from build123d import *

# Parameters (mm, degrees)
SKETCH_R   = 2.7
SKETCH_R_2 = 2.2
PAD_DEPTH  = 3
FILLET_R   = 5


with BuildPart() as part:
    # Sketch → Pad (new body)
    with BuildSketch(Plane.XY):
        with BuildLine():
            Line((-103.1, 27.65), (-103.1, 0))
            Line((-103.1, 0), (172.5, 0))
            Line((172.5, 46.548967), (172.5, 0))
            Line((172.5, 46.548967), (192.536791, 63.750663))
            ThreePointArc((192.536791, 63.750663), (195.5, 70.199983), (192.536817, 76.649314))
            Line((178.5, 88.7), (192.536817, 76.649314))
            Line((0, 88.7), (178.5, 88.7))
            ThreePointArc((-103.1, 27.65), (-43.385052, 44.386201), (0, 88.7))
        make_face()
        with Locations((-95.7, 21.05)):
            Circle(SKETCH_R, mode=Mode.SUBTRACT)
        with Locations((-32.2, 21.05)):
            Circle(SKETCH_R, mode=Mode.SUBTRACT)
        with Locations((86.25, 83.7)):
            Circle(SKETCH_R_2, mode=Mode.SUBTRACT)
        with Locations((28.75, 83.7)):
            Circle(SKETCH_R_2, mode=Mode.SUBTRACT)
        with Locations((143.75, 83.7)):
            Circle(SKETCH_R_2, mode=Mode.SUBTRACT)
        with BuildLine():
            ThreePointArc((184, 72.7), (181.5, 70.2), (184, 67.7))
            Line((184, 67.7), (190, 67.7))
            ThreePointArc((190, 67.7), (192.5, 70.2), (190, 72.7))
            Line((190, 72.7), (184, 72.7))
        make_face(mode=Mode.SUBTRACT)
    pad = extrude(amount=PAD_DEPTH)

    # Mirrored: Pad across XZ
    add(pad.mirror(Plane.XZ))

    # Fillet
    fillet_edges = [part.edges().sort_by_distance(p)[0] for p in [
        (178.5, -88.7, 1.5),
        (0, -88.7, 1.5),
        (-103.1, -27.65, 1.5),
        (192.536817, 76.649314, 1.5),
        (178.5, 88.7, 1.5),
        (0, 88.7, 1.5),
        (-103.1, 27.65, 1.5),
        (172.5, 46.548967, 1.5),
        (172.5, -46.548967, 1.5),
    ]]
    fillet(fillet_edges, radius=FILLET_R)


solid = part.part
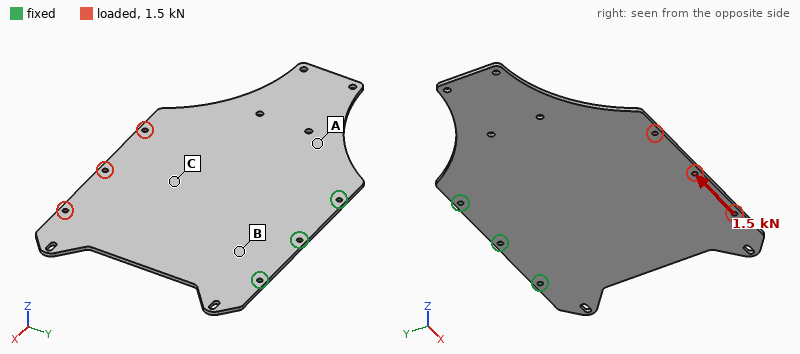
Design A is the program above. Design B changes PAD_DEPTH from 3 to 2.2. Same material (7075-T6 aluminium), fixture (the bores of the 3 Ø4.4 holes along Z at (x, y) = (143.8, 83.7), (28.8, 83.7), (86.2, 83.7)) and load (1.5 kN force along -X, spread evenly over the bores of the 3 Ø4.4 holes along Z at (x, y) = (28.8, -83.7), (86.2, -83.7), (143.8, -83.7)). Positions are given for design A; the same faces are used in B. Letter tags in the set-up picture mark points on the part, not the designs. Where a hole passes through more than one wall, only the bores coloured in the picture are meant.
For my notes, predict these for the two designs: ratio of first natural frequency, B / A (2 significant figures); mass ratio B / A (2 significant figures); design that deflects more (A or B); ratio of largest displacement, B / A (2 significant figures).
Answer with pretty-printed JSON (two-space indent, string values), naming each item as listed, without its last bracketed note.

{
  "ratio of first natural frequency, B / A": "0.74",
  "mass ratio B / A": "0.73",
  "design that deflects more": "B",
  "ratio of largest displacement, B / A": "1.4"
}
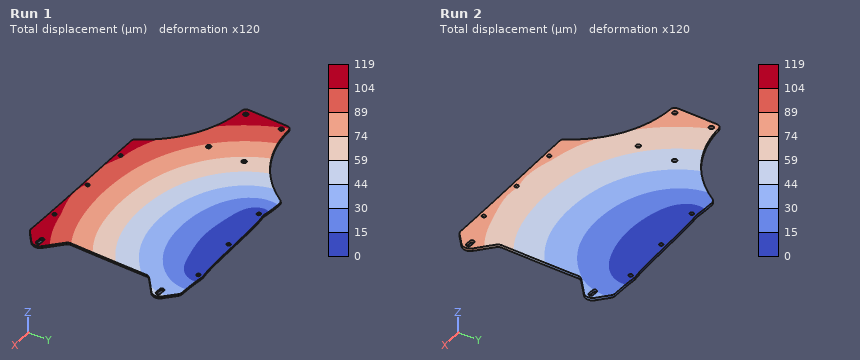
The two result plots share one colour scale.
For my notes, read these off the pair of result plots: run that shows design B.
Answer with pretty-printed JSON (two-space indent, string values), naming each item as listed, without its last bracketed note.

{
  "run that shows design B": "Run 1"
}
